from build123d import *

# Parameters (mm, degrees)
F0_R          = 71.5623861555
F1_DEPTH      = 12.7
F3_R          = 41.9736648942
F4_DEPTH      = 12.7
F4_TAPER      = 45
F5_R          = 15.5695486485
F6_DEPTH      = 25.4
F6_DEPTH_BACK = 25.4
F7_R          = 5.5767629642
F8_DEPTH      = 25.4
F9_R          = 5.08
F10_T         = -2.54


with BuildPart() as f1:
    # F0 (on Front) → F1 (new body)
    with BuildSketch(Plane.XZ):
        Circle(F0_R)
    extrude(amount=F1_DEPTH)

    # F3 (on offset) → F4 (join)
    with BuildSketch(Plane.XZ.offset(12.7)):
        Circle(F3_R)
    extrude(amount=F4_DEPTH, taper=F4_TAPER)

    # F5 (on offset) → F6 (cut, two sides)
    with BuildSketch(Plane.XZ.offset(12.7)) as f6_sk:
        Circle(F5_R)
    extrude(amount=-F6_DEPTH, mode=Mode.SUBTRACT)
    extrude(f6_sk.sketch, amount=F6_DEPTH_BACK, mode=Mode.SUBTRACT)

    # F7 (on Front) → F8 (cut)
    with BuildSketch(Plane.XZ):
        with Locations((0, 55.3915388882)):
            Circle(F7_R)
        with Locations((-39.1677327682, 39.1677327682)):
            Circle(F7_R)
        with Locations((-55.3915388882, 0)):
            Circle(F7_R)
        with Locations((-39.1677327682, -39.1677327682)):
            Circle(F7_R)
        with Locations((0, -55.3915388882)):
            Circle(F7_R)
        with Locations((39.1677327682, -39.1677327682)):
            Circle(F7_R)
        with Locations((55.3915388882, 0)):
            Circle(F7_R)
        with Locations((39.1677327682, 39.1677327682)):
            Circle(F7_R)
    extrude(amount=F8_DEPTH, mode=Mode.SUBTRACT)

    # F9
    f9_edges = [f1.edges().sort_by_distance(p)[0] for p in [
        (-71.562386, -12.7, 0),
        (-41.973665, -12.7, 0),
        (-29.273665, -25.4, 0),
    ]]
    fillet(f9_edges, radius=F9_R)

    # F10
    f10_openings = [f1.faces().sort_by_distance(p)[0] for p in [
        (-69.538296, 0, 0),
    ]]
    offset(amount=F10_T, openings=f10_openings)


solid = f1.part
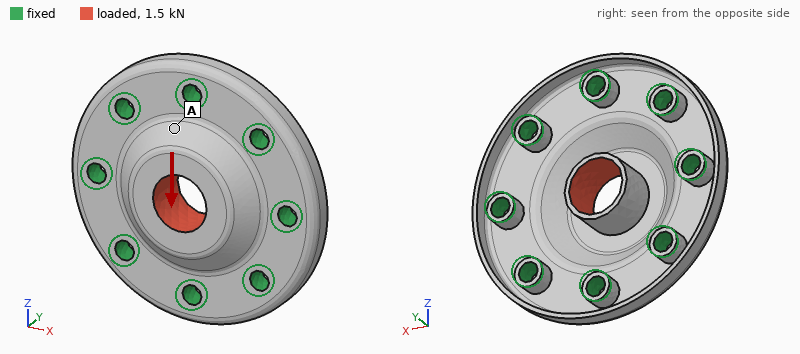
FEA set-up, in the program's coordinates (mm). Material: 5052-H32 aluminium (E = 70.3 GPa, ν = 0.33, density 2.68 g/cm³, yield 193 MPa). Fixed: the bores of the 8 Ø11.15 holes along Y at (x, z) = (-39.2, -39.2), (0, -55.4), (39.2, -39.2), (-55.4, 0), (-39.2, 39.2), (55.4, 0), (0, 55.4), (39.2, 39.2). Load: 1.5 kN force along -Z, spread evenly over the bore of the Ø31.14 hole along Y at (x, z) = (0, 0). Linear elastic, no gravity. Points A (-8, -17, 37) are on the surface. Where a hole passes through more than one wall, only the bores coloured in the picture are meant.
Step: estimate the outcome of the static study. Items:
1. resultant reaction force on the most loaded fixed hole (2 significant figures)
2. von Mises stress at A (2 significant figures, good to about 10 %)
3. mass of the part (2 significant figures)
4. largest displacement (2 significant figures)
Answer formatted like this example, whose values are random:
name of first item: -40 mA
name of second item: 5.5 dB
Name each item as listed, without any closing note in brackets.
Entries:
resultant reaction force on the most loaded fixed hole: 280 N
von Mises stress at A: 6.5 MPa
mass of the part: 170 g
largest displacement: 75 µm
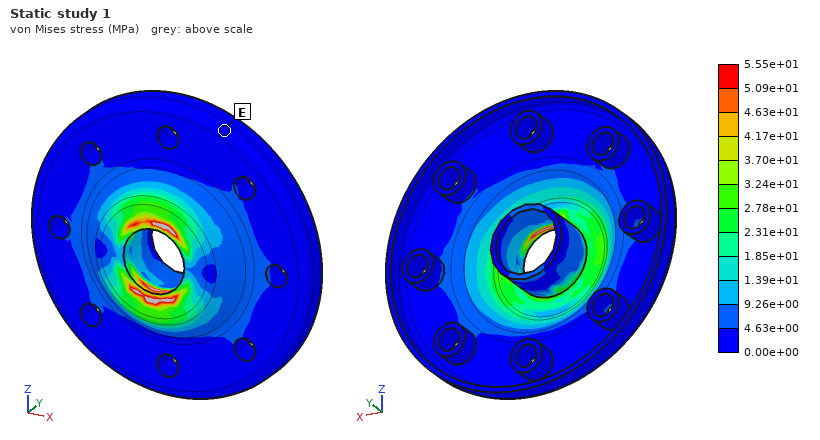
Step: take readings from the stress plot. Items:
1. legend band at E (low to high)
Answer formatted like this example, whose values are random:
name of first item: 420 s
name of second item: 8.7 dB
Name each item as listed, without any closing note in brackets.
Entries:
legend band at E: 0.00e+00 to 4.63e+00 MPa
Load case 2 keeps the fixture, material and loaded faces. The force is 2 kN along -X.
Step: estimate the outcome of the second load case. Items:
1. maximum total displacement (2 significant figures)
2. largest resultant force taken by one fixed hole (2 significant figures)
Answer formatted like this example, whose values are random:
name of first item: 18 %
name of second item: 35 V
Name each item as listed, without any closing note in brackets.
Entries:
maximum total displacement: 0.10 mm
largest resultant force taken by one fixed hole: 370 N
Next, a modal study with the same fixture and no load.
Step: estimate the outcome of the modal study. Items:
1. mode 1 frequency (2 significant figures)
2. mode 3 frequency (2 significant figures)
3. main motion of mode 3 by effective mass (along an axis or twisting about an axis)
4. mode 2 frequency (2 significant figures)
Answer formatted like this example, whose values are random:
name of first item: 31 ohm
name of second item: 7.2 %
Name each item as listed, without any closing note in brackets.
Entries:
mode 1 frequency: 5300 Hz
mode 3 frequency: 5600 Hz
main motion of mode 3 by effective mass: along Y
mode 2 frequency: 5300 Hz
